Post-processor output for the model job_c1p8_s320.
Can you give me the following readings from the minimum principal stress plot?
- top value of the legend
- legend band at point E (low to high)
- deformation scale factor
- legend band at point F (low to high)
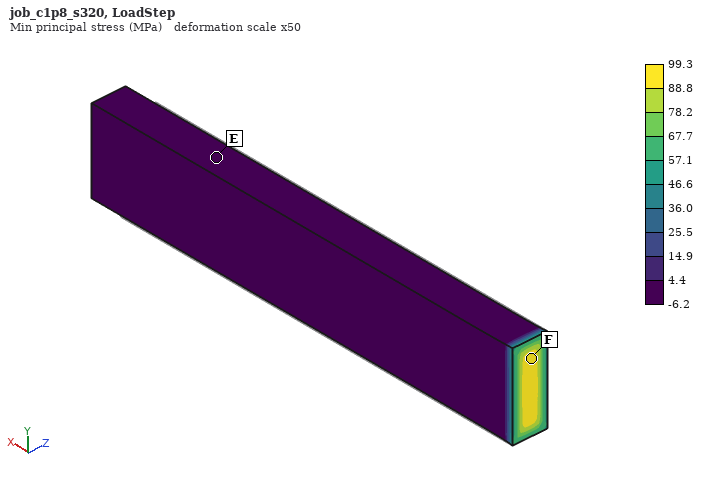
99.3 MPa
-6.2 to 4.4 MPa
50
88.8 to 99.3 MPa
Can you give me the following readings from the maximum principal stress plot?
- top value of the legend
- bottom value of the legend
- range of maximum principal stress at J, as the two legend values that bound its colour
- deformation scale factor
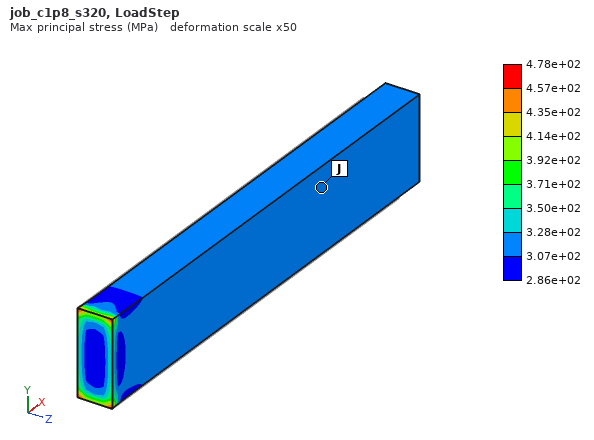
4.78e+02 MPa
2.86e+02 MPa
3.07e+02 to 3.28e+02 MPa
50
